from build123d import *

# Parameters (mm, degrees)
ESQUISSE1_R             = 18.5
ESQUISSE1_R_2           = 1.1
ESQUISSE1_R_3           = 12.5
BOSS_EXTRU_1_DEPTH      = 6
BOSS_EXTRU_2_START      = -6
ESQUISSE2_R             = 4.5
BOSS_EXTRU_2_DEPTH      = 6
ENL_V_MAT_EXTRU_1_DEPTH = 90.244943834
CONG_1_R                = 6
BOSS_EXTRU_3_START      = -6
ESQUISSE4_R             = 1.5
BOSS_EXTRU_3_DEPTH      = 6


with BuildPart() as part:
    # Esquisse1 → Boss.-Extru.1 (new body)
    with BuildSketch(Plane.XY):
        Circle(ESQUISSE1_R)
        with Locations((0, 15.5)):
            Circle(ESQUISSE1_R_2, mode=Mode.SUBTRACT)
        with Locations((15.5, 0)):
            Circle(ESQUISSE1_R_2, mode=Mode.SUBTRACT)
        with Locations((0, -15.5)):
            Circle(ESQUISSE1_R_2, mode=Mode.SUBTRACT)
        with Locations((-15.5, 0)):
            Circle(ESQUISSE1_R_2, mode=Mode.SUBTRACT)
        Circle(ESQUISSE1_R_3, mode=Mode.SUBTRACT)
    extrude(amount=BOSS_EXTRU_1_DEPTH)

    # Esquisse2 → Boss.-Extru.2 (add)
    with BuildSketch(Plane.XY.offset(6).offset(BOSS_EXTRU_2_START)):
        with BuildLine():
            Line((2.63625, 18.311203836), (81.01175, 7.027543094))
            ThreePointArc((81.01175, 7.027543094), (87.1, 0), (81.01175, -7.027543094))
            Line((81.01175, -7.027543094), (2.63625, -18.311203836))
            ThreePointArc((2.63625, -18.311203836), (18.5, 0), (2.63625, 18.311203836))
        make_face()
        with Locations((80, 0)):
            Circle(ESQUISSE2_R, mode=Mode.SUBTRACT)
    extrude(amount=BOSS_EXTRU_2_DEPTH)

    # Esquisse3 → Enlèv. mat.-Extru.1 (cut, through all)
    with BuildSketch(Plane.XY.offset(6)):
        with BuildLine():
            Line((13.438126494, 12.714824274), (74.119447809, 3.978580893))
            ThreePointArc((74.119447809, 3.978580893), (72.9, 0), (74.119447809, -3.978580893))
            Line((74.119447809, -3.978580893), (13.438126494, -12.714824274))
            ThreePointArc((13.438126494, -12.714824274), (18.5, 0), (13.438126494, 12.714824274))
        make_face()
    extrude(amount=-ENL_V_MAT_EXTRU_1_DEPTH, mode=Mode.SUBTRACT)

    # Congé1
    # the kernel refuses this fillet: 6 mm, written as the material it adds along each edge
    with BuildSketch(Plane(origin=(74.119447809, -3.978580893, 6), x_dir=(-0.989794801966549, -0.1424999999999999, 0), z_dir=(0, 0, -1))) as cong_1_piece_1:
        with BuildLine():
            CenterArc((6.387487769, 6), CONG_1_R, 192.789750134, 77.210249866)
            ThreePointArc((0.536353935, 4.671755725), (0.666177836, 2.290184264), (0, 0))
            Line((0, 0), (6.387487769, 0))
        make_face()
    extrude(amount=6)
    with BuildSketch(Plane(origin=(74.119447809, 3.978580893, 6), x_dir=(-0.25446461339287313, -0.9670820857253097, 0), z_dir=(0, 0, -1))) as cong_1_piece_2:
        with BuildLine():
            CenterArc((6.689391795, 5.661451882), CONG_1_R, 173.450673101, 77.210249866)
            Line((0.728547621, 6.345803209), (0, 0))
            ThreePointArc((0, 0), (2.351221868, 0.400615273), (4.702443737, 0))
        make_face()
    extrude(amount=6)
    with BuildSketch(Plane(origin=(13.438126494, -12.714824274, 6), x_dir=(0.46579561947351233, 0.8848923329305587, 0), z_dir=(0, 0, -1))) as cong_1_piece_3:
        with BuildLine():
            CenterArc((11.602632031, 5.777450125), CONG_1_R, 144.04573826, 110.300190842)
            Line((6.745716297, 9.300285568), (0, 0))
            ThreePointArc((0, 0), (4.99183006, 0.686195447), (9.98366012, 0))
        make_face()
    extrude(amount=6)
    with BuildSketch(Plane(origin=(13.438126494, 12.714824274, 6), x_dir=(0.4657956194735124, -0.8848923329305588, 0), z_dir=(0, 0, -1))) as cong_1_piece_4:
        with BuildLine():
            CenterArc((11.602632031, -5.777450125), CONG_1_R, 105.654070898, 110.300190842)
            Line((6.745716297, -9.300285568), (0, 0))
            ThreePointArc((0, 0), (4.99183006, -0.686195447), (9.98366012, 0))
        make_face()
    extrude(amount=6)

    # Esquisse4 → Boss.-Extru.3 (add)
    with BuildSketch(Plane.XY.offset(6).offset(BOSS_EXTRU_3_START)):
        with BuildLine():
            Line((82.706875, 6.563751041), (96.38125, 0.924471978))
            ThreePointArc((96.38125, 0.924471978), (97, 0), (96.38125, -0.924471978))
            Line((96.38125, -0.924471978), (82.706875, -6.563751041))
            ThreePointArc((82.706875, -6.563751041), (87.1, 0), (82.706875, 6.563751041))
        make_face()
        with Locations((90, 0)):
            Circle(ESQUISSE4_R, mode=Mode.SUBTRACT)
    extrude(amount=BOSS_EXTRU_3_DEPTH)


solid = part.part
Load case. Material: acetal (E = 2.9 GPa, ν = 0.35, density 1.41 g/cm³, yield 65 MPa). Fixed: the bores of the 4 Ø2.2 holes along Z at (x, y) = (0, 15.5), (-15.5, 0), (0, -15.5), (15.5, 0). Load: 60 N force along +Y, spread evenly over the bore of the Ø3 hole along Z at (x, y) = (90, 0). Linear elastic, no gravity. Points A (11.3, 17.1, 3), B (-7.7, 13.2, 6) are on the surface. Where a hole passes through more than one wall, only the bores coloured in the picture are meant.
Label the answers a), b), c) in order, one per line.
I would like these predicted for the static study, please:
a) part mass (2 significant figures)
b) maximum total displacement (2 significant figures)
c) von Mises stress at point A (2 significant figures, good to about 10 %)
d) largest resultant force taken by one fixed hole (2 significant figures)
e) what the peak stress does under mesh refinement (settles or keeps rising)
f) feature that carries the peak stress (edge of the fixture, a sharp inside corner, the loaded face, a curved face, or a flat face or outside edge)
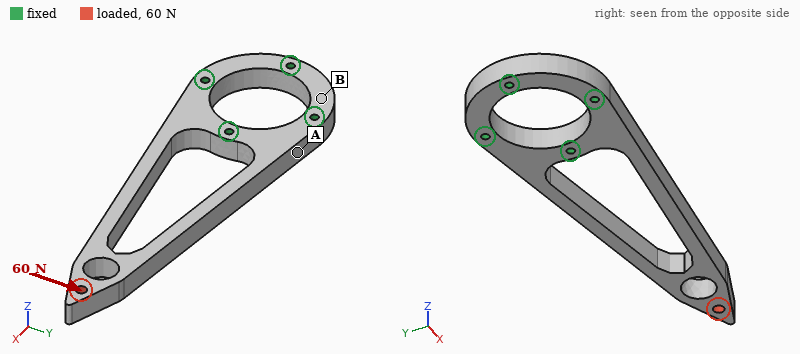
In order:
a) 11 g
b) 1.4 mm
c) 7.4 MPa
d) 150 N
e) keeps rising
f) a sharp inside corner
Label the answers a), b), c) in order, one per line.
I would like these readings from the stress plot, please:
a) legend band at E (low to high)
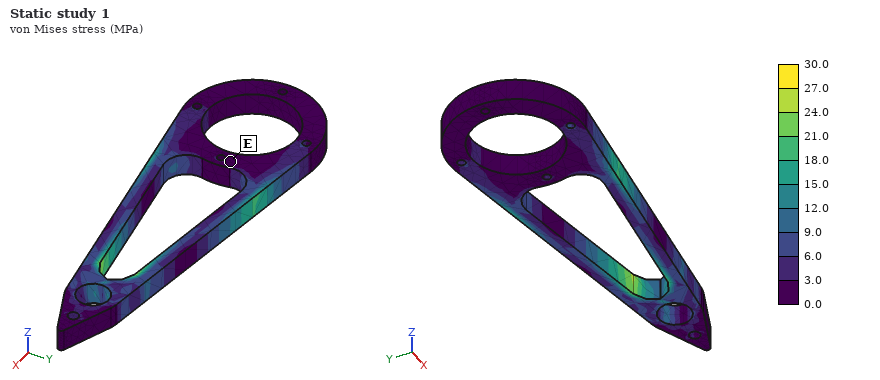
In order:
a) 0.0 to 3.0 MPa
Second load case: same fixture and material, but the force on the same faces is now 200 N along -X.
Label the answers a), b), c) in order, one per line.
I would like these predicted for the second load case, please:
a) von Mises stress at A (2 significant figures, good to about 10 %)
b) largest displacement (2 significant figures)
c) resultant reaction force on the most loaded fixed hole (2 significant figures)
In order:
a) 4.0 MPa
b) 0.14 mm
c) 92 N
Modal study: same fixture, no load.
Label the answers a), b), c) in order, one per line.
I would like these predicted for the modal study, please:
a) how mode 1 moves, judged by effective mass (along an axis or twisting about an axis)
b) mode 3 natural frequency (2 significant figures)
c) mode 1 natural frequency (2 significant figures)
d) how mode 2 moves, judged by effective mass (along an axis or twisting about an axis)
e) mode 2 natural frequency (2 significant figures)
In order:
a) along Z
b) 990 Hz
c) 210 Hz
d) along Y
e) 530 Hz
